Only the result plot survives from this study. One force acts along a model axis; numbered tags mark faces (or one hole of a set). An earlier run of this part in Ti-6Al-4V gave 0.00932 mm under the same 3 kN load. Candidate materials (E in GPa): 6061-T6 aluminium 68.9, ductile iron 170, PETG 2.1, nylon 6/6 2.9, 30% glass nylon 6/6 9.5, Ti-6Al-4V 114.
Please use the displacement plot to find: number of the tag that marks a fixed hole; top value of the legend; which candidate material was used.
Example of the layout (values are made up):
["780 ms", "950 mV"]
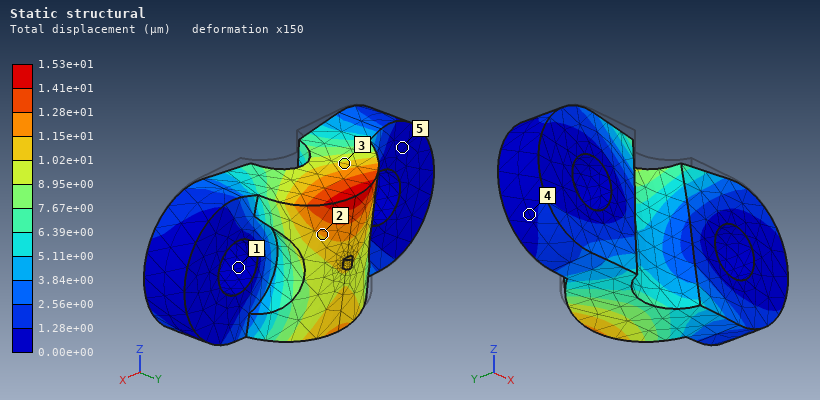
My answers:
["1", "1.53e+01 µm", "6061-T6 aluminium"]
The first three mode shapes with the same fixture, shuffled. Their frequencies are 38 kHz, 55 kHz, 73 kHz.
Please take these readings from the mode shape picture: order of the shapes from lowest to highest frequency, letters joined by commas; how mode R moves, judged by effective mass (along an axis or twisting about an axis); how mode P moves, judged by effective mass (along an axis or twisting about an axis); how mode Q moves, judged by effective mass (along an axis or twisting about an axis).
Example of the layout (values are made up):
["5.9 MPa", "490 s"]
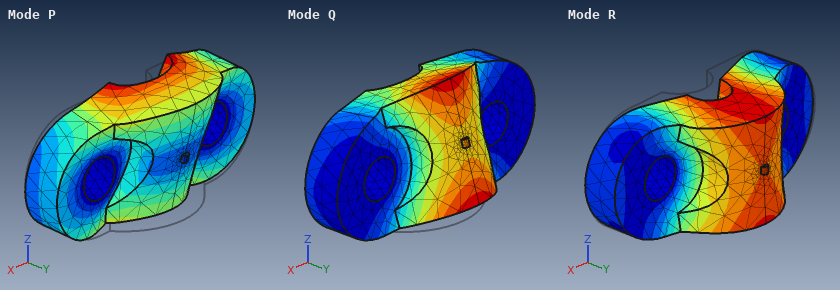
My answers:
["Q, R, P", "along Y", "along Z", "along Z"]
